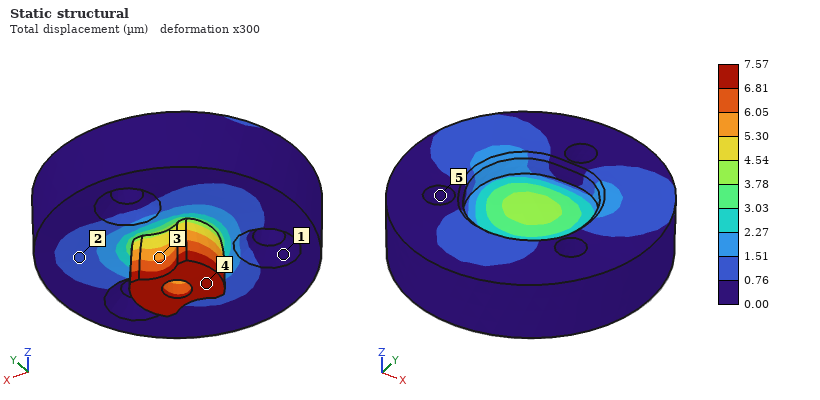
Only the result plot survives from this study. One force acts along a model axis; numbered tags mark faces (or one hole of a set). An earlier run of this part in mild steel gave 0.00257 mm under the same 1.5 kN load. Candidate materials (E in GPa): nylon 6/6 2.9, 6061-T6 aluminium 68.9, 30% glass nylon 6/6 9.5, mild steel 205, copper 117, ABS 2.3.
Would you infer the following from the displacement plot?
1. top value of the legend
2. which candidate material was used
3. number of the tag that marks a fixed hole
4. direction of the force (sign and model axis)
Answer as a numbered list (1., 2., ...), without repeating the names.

1. 7.57 µm
2. 6061-T6 aluminium
3. 5
4. +Z
